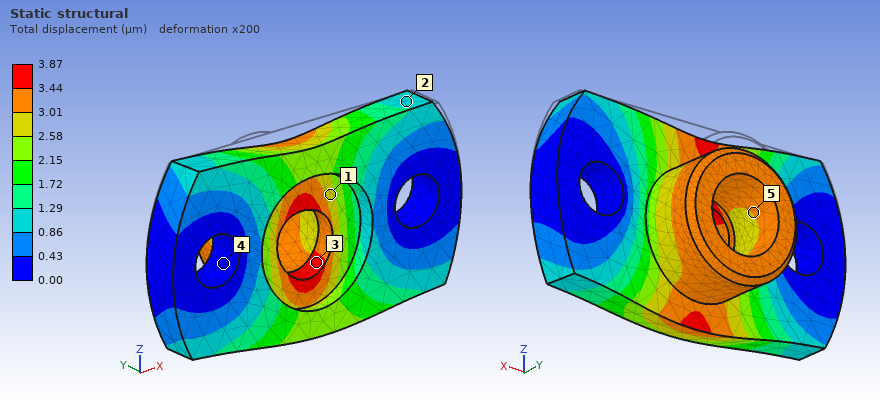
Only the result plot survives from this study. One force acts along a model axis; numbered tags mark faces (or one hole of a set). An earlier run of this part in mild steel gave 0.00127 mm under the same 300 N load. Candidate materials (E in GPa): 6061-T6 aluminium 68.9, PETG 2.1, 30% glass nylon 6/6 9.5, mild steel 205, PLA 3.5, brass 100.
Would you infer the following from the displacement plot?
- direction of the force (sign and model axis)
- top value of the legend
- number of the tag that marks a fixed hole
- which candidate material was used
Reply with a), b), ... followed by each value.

a) -Z
b) 3.87 µm
c) 4
d) 6061-T6 aluminium
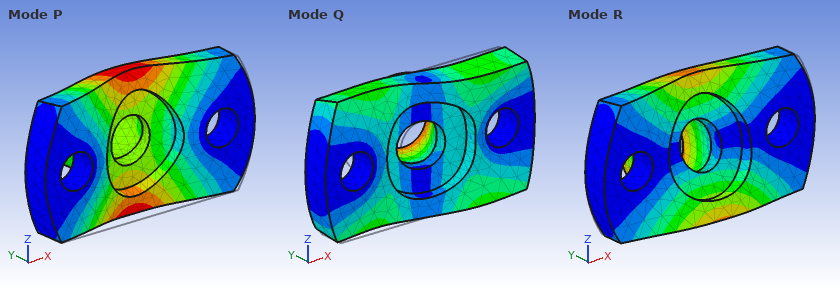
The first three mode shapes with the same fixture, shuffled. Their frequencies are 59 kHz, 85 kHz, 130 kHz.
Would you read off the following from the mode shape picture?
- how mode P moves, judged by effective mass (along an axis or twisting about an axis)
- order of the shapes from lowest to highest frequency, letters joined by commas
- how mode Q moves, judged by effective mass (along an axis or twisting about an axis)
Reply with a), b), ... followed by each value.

a) along Y
b) R, P, Q
c) along X
